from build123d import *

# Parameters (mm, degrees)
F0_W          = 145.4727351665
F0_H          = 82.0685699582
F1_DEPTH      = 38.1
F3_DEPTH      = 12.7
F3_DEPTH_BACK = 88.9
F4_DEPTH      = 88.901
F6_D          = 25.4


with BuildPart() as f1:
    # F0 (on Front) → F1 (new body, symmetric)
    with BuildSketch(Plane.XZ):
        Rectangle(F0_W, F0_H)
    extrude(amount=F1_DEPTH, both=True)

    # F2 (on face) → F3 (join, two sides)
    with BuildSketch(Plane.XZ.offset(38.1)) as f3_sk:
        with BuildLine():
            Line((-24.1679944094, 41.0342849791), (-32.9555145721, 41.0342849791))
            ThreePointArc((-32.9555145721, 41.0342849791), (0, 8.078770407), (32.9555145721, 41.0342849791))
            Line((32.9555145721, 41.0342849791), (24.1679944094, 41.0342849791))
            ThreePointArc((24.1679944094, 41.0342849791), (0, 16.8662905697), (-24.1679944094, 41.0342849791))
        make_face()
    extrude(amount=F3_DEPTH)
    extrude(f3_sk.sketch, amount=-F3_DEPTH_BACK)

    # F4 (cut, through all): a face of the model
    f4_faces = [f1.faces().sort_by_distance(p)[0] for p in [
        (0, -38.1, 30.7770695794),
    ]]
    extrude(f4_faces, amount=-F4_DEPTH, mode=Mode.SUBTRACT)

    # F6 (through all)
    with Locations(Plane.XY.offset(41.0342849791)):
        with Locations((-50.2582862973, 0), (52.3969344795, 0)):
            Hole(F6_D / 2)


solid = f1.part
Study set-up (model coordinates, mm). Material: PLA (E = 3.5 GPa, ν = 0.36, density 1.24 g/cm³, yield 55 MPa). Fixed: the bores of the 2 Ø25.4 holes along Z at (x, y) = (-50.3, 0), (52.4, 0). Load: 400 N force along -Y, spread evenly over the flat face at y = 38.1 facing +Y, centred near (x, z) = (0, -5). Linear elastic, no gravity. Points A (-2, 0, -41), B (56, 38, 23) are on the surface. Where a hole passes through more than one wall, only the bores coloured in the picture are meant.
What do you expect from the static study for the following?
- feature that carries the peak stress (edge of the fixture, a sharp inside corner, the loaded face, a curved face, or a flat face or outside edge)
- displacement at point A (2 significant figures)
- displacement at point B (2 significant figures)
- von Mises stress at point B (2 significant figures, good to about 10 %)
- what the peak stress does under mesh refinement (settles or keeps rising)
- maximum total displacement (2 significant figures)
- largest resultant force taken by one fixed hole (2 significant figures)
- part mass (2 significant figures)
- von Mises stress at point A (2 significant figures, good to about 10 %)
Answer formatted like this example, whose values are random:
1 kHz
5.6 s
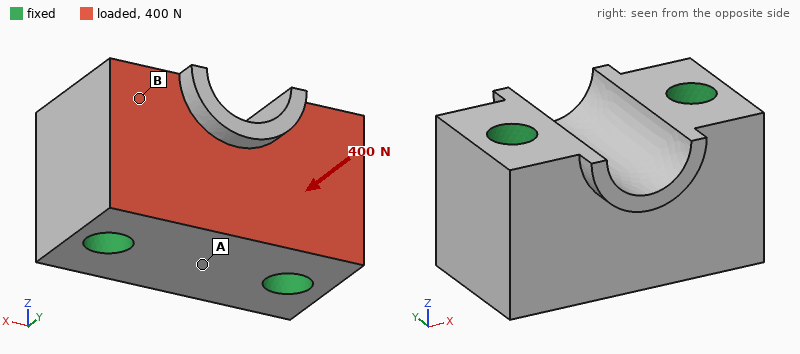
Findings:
edge of the fixture
0.60 µm
0.32 µm
0.045 MPa
keeps rising
0.96 µm
200 N
960 g
0.019 MPa
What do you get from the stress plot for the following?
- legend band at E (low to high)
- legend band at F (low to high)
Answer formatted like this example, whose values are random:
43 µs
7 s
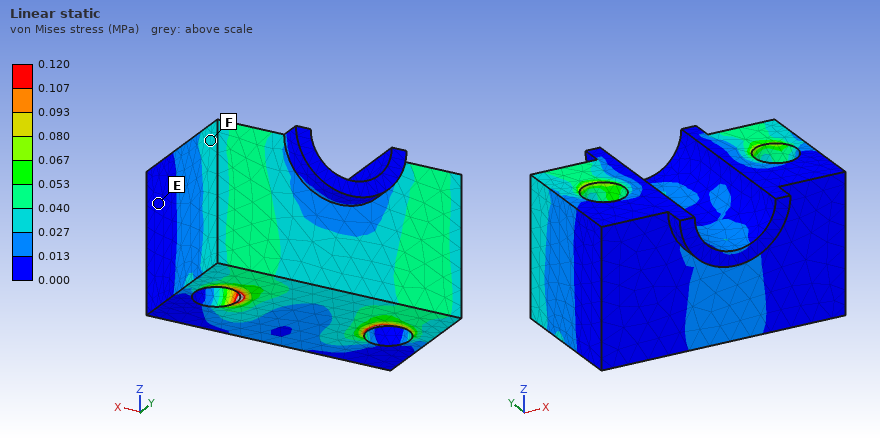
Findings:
0.000 to 0.013 MPa
0.027 to 0.040 MPa
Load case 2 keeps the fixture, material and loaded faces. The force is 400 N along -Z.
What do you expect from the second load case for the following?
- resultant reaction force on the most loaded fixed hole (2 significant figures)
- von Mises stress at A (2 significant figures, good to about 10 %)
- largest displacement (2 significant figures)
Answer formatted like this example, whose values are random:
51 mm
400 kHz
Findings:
200 N
0.040 MPa
2.5 µm
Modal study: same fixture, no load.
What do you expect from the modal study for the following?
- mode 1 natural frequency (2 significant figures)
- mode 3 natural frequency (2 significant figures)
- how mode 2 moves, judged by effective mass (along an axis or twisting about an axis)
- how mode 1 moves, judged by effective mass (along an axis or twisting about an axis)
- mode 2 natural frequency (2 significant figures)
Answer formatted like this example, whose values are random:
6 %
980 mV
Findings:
4500 Hz
5100 Hz
along Z
along Y
4700 Hz
